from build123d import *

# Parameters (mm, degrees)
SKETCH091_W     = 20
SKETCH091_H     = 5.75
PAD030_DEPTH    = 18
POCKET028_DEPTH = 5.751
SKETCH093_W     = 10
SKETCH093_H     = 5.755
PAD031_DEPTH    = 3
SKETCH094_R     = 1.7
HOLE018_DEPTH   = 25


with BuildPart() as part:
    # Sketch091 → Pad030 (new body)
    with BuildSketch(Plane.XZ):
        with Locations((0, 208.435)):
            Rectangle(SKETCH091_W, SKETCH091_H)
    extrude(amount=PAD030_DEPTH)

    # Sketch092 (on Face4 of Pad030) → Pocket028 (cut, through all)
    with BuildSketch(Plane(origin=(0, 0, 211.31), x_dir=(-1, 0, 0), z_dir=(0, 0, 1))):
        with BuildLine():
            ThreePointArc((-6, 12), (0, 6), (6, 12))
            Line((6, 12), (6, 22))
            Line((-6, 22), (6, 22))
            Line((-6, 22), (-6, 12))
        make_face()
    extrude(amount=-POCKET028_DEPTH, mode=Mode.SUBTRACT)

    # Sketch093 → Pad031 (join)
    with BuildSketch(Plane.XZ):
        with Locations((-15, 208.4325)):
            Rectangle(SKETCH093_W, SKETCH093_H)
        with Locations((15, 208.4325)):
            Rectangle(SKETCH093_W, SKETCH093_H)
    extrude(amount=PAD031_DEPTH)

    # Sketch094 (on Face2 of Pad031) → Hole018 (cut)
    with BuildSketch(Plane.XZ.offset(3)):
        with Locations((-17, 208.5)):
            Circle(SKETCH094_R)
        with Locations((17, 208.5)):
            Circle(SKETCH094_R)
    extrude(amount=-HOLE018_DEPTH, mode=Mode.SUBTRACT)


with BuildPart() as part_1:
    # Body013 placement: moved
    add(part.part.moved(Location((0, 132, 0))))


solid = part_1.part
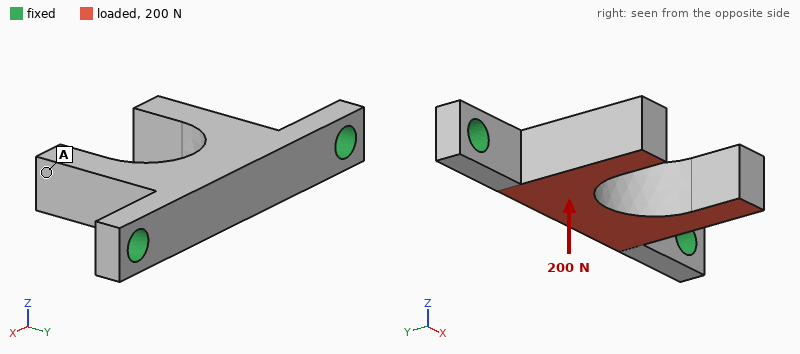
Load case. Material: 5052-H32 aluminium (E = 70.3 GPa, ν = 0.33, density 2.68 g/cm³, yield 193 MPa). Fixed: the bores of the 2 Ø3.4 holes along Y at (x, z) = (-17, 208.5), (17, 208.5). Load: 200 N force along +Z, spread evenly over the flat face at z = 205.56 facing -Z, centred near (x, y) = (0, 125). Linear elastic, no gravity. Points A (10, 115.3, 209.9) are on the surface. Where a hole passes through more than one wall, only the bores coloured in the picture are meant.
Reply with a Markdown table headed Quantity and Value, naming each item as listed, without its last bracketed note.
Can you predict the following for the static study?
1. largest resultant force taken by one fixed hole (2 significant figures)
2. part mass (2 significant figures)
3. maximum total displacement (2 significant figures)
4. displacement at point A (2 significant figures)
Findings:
| Quantity | Value |
|---|---|
| largest resultant force taken by one fixed hole | 100 N |
| part mass | 4.3 g |
| maximum total displacement | 72 µm |
| displacement at point A | 65 µm |
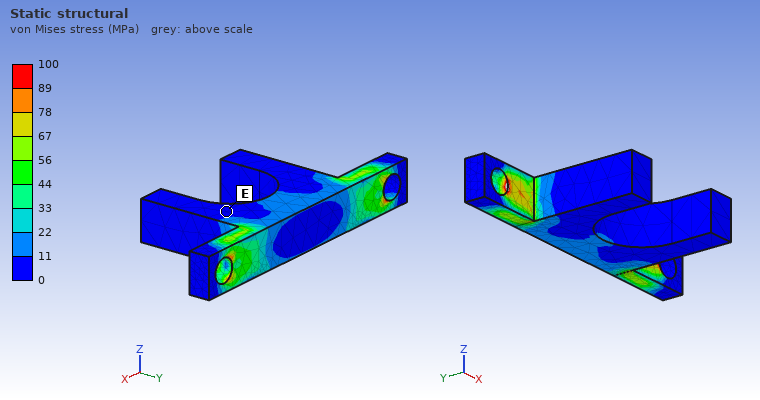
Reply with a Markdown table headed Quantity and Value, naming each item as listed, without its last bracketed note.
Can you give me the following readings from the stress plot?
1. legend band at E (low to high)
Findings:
| Quantity | Value |
|---|---|
| legend band at E | 0 to 11 MPa |
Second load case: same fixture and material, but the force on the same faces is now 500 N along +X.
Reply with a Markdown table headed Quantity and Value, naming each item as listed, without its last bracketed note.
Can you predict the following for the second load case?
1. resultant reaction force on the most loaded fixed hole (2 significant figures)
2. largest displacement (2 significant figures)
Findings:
| Quantity | Value |
|---|---|
| resultant reaction force on the most loaded fixed hole | 280 N |
| largest displacement | 21 µm |
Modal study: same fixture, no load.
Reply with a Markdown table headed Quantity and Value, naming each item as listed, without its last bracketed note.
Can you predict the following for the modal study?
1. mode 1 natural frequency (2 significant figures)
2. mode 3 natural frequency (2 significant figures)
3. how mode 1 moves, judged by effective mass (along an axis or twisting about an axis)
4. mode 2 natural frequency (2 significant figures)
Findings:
| Quantity | Value |
|---|---|
| mode 1 natural frequency | 5700 Hz |
| mode 3 natural frequency | 14 kHz |
| how mode 1 moves, judged by effective mass | along Z |
| mode 2 natural frequency | 14 kHz |
